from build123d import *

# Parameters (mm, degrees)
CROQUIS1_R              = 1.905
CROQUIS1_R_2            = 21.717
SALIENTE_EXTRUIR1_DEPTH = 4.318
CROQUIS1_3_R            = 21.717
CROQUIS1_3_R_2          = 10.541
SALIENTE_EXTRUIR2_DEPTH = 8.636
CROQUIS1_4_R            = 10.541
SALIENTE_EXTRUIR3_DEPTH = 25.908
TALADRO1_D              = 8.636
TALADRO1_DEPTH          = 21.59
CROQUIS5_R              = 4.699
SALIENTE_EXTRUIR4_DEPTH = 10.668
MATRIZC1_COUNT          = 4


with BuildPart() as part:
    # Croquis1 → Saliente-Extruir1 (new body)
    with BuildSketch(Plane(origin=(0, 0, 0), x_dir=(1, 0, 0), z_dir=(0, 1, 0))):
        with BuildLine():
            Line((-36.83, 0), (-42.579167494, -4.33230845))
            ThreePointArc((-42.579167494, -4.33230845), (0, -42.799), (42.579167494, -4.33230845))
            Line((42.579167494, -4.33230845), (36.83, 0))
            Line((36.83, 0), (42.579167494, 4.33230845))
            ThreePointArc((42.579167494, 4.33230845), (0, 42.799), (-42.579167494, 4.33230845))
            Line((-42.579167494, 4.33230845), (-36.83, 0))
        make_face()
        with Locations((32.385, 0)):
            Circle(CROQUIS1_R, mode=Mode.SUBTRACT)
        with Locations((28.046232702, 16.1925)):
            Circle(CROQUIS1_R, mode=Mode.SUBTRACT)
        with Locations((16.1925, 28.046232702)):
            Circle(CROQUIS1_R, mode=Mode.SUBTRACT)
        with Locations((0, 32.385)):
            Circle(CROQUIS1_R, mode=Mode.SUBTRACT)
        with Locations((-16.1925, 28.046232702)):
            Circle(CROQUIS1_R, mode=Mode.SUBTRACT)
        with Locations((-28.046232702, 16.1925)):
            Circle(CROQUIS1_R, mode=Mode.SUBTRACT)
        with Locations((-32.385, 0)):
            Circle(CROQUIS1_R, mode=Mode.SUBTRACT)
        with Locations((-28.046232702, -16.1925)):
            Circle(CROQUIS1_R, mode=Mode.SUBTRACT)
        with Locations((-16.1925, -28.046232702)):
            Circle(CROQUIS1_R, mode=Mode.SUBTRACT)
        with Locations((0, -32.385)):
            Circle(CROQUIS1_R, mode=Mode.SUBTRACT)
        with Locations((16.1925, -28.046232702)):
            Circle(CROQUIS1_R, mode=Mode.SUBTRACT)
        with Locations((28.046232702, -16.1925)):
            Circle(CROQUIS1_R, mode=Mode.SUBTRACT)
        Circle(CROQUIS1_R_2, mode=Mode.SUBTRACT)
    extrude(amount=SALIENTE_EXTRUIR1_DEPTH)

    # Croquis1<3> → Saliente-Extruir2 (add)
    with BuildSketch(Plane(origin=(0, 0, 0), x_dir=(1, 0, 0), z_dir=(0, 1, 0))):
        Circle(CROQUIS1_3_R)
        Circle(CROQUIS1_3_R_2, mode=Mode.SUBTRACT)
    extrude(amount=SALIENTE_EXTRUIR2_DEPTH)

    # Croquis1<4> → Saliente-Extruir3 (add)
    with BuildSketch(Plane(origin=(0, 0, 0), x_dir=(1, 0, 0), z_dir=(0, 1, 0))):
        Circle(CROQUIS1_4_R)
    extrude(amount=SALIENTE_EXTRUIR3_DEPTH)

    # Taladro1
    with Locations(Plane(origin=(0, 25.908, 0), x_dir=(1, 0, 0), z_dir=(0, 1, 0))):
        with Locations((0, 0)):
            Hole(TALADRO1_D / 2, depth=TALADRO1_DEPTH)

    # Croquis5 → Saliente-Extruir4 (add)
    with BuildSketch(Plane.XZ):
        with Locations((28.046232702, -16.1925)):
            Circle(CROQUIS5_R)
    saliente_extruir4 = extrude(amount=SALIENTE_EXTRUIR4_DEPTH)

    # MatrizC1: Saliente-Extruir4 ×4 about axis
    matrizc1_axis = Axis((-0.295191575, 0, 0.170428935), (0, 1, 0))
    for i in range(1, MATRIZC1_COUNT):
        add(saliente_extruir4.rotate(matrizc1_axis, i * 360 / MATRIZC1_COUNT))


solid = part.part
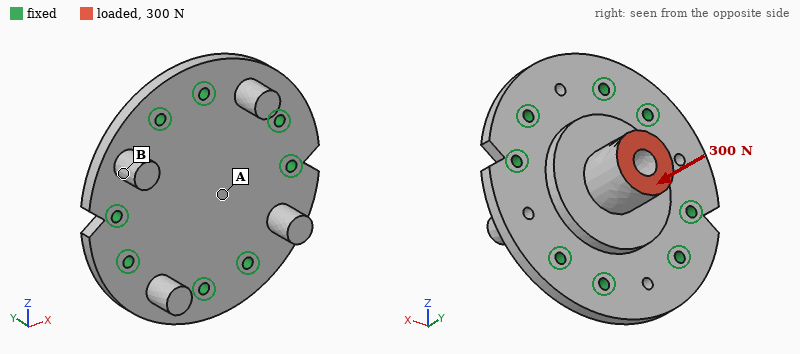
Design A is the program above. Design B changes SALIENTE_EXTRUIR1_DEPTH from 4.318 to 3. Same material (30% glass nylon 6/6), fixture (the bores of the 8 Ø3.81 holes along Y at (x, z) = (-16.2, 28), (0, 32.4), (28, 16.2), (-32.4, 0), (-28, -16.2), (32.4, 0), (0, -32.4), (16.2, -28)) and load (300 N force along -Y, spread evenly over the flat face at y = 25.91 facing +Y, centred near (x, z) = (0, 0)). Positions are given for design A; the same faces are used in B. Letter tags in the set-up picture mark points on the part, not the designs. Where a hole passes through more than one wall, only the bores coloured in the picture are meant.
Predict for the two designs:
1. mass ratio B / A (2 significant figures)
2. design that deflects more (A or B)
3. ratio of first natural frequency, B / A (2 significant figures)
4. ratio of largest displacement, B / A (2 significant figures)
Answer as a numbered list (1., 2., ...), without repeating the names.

1. 0.86
2. B
3. 0.76
4. 1.5
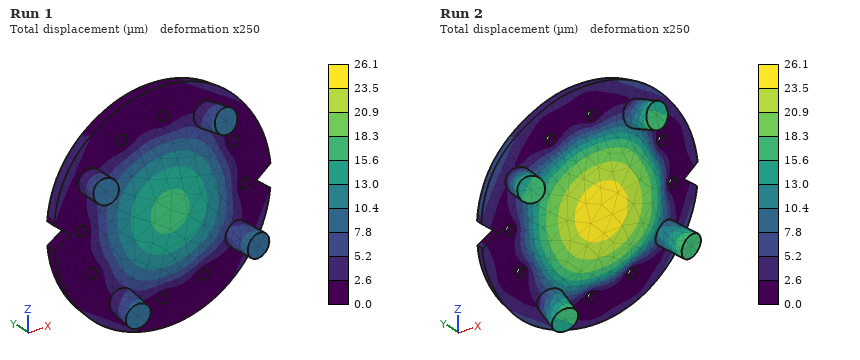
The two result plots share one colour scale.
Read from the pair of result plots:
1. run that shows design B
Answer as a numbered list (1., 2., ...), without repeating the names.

1. Run 2
